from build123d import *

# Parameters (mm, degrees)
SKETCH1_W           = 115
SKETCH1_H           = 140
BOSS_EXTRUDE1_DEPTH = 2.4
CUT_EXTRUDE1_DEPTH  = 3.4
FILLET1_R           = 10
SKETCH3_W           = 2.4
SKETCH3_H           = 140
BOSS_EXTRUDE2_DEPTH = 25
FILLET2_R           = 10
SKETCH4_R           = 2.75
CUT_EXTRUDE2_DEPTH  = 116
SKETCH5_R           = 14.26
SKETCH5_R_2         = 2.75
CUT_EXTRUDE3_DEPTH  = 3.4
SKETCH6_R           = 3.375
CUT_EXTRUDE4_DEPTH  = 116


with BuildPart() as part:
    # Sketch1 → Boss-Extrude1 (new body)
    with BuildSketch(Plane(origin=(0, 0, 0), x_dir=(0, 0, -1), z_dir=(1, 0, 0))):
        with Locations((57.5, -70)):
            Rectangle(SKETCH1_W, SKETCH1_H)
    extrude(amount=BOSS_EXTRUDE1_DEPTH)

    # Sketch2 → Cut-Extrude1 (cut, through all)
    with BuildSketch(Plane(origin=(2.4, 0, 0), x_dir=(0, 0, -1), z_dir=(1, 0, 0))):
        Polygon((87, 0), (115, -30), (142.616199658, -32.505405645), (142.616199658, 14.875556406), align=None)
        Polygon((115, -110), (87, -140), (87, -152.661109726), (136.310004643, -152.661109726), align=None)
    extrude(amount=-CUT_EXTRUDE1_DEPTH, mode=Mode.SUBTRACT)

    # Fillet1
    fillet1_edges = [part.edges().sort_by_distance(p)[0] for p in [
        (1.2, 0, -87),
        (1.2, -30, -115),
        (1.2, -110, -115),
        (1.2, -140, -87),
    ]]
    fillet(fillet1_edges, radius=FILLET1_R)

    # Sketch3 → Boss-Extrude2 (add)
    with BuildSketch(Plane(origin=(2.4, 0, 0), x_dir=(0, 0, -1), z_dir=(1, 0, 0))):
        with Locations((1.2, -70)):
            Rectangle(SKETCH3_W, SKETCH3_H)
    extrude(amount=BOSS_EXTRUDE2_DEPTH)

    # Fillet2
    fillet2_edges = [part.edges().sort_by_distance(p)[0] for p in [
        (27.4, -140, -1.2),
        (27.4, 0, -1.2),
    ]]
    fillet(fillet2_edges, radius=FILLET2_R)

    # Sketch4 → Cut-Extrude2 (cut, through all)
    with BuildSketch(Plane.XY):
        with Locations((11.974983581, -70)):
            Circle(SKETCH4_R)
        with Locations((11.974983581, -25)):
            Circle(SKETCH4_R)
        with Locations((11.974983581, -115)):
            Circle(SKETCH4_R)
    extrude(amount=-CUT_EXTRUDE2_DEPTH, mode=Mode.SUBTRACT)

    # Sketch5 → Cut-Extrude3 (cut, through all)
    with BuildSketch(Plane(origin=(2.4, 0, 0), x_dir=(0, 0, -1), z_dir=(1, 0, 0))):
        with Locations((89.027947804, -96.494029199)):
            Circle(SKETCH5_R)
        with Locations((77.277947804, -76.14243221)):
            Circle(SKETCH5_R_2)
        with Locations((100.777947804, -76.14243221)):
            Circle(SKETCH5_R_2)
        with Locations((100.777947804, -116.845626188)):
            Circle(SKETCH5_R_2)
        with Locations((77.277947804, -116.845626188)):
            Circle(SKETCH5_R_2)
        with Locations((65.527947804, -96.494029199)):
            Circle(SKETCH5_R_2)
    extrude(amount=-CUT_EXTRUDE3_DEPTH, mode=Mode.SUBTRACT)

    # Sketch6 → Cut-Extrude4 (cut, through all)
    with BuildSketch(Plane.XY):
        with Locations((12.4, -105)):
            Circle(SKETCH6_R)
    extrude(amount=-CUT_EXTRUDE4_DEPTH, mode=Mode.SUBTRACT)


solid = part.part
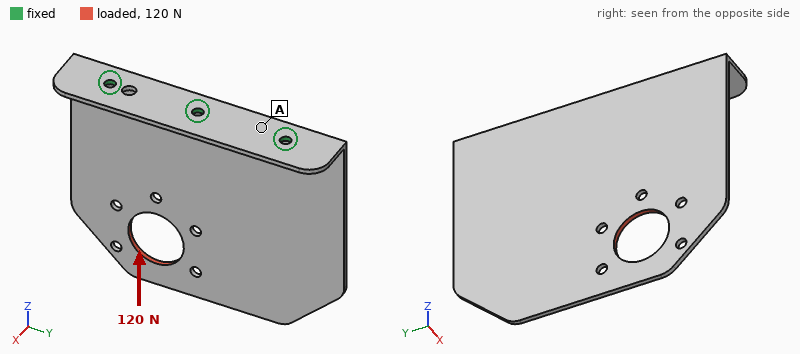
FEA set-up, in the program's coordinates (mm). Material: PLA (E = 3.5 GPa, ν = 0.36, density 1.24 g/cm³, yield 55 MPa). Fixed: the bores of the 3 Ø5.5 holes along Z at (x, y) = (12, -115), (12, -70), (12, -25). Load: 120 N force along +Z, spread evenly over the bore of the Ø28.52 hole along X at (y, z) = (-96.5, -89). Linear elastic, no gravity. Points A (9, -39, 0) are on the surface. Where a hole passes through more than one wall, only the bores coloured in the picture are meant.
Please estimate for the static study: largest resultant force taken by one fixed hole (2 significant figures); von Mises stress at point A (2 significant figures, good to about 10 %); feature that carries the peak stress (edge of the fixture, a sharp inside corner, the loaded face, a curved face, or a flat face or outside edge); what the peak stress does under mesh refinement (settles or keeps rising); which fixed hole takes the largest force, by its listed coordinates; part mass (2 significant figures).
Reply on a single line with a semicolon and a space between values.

74 N; 1.6 MPa; edge of the fixture; keeps rising; (12, -115); 53 g
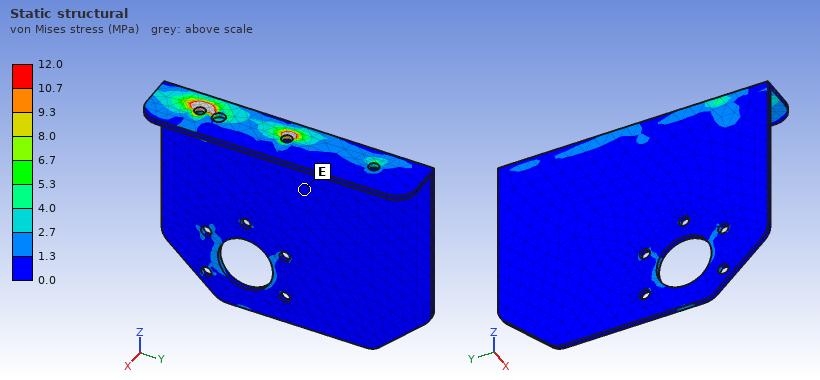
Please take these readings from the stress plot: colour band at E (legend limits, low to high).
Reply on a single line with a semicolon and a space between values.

0.0 to 1.3 MPa
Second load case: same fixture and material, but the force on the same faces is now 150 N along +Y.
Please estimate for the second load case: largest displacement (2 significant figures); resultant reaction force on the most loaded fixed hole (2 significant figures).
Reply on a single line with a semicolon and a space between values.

1.8 mm; 150 N
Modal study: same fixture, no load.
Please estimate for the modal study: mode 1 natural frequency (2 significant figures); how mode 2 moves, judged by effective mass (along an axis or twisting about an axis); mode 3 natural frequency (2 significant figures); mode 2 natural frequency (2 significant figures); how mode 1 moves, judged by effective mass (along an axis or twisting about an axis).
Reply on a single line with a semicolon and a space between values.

51 Hz; twisting about Z; 260 Hz; 120 Hz; along X
